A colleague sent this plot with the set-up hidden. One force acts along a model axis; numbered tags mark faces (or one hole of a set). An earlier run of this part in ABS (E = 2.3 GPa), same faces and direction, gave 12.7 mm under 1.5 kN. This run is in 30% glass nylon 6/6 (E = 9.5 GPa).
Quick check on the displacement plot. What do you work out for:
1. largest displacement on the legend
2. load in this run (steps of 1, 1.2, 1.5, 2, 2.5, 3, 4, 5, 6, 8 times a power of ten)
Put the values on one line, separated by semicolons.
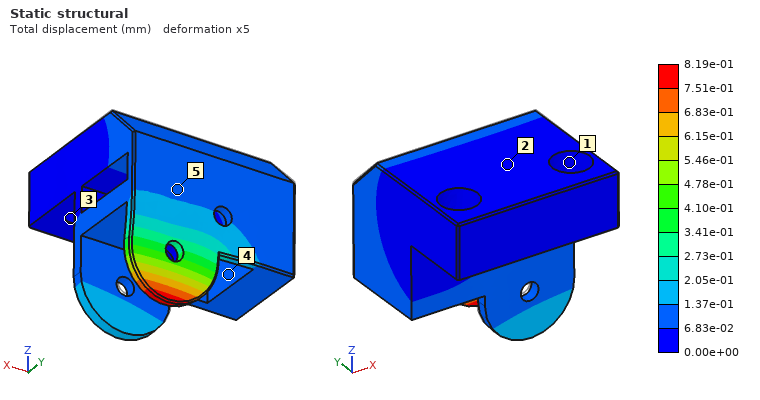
8.19e-01 mm; 400 N
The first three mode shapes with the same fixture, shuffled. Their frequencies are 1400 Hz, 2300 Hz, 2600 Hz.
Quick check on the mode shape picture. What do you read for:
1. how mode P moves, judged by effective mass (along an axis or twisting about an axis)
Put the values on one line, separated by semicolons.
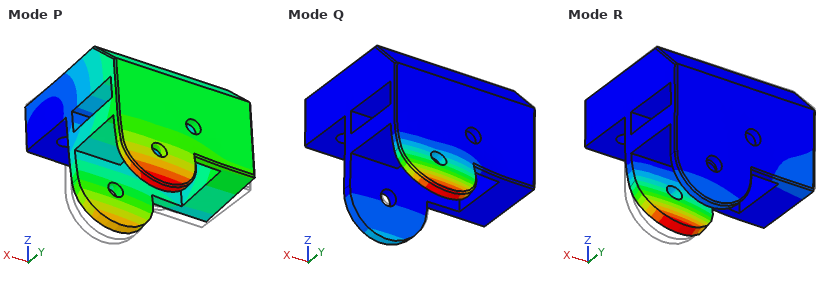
along Z
